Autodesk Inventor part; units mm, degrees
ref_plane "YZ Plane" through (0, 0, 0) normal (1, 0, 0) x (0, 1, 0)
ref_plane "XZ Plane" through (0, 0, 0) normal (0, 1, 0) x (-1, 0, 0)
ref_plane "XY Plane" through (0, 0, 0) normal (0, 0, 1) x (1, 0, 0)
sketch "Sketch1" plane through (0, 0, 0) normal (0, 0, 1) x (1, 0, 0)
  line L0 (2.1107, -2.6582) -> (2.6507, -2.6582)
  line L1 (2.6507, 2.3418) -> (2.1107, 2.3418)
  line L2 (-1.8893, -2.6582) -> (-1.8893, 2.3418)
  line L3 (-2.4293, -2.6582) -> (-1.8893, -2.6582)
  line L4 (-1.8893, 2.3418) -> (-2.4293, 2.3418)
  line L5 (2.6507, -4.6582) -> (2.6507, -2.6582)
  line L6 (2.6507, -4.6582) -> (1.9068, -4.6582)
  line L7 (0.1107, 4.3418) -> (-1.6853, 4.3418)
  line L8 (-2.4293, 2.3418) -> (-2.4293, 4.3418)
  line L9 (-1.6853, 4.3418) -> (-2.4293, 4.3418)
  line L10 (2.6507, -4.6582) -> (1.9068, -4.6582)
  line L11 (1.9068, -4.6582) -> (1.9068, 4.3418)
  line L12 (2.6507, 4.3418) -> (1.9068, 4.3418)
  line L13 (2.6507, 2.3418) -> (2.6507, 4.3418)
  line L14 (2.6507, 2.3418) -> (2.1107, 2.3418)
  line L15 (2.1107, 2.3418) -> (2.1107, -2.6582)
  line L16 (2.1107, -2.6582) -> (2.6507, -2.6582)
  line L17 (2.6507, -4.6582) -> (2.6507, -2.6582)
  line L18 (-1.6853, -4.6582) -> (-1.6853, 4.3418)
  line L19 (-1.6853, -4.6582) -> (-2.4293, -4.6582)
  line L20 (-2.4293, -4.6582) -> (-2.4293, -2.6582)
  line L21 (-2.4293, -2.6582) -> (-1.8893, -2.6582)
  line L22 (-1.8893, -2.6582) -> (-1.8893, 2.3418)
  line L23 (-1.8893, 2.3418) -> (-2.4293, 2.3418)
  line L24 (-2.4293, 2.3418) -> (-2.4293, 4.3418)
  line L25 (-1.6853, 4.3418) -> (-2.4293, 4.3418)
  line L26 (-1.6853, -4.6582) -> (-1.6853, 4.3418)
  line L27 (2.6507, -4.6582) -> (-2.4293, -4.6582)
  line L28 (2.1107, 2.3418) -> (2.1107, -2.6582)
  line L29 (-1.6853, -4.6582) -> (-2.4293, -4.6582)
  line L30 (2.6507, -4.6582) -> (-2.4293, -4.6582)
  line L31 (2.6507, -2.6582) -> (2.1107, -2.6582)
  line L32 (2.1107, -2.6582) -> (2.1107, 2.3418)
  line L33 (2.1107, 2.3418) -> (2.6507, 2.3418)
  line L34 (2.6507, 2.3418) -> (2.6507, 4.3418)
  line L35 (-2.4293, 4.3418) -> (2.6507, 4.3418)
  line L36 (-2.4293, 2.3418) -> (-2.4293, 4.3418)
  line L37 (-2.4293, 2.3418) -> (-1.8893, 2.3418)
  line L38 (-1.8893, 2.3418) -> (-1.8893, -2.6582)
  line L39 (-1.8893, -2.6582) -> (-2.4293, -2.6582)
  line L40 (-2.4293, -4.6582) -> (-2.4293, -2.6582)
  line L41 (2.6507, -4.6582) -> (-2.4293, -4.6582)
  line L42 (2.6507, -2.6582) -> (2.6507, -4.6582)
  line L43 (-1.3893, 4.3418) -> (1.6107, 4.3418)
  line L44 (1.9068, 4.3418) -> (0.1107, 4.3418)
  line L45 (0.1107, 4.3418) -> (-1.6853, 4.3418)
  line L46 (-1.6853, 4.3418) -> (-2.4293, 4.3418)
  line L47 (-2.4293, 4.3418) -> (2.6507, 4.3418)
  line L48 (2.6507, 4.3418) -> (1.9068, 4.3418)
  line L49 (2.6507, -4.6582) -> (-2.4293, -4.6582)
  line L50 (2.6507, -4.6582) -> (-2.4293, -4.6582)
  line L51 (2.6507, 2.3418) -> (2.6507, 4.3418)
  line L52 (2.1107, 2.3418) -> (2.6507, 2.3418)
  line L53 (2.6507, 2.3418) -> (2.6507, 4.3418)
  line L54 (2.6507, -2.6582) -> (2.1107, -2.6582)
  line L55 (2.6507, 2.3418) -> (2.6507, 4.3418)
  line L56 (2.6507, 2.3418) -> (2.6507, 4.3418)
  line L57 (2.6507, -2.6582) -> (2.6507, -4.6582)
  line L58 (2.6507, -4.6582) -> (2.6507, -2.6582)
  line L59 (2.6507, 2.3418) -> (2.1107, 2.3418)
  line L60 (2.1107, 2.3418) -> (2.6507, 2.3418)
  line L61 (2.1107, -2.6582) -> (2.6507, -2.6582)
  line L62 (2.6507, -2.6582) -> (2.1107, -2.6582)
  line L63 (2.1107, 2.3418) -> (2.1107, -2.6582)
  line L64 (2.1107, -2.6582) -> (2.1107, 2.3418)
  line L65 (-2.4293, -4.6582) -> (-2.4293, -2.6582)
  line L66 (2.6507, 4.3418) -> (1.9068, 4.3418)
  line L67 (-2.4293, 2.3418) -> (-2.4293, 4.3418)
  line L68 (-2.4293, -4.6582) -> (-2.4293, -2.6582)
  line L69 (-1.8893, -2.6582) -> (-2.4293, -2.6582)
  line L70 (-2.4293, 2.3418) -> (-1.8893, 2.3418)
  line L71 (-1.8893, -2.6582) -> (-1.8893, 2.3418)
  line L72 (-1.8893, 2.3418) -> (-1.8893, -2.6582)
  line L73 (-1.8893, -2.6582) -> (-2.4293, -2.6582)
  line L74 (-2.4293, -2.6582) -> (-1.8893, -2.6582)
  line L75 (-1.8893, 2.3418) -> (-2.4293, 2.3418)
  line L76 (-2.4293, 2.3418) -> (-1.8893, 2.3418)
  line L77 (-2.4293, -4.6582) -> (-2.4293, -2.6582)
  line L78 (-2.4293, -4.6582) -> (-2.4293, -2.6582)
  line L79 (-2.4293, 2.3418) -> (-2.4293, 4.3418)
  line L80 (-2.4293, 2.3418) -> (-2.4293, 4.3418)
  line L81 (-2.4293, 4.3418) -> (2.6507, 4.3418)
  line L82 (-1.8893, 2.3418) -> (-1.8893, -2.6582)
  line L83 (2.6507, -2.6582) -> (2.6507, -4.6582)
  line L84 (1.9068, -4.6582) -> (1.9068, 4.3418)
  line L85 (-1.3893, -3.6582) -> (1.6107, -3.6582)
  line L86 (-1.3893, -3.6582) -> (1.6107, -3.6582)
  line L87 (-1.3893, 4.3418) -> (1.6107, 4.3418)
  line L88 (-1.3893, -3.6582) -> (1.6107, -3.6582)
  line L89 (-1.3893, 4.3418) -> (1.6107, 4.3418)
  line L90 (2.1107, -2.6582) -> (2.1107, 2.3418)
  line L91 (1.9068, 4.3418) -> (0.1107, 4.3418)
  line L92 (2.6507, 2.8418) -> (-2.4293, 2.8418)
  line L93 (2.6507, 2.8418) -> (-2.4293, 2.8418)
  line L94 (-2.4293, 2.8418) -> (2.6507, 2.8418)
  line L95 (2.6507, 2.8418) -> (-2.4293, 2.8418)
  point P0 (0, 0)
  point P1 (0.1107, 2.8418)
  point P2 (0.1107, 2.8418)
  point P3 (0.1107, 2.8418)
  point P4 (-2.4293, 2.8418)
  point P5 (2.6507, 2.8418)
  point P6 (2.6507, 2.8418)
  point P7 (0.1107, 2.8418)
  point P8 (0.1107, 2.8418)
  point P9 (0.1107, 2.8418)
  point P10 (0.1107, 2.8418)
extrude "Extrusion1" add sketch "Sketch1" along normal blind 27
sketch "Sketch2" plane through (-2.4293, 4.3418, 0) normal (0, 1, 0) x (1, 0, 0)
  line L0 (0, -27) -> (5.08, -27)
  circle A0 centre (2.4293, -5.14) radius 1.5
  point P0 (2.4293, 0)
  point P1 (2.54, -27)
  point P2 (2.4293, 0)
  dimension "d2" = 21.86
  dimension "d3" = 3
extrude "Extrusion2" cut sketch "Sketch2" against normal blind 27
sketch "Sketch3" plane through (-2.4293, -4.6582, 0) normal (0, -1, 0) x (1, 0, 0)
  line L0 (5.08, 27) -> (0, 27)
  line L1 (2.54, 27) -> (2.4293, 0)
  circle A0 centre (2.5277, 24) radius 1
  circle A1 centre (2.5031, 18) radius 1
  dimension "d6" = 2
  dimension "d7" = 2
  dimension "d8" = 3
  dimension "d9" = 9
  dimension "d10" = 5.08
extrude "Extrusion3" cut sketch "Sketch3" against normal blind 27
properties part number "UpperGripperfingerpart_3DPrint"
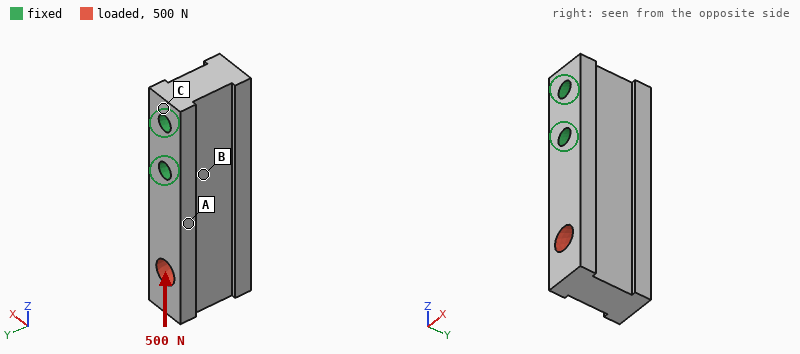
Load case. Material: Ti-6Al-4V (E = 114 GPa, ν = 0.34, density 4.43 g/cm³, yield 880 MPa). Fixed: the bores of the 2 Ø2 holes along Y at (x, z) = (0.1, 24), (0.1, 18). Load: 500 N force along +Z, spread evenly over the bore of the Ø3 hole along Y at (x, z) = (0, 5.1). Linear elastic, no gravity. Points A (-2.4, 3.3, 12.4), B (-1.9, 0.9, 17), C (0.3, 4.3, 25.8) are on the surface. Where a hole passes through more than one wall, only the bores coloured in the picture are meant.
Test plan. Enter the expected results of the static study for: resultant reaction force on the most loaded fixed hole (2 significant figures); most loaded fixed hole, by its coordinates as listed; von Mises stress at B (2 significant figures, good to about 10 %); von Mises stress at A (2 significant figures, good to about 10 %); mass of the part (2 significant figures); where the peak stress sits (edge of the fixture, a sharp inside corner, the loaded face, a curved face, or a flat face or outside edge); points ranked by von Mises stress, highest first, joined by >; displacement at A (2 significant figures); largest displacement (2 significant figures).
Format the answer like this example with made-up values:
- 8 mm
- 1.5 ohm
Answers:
- 470 N
- (0.1, 18)
- 7.5 MPa
- 14 MPa
- 4.3 g
- the loaded face
- A > B > C
- 0.72 µm
- 2.5 µm
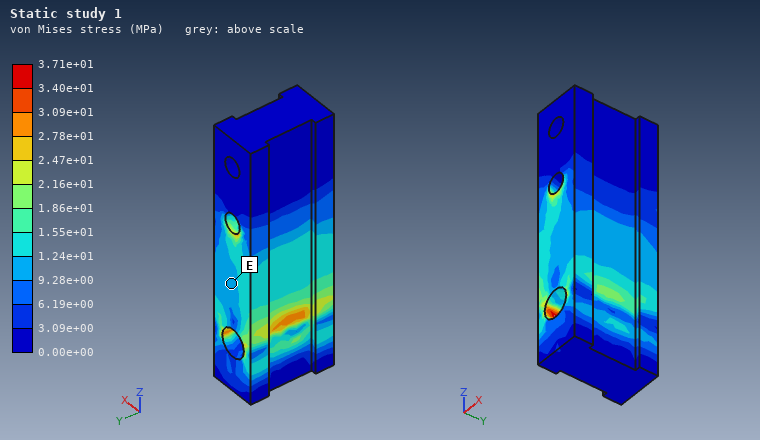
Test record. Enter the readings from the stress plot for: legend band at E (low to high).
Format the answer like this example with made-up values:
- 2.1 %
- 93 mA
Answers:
- 9.28e+00 to 1.24e+01 MPa
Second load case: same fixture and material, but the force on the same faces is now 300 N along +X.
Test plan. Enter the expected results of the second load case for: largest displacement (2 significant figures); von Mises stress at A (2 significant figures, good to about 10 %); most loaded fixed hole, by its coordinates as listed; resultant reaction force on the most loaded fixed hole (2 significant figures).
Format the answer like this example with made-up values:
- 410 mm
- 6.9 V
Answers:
- 52 µm
- 78 MPa
- (0.1, 18)
- 480 N
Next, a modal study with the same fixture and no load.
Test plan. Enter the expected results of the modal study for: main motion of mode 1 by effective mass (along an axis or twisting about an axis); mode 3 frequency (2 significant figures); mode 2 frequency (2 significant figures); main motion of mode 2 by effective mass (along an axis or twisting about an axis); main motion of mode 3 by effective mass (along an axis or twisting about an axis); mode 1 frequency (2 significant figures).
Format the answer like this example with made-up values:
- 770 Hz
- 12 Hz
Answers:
- along X
- 31 kHz
- 21 kHz
- along Y
- twisting about Z
- 11 kHz
